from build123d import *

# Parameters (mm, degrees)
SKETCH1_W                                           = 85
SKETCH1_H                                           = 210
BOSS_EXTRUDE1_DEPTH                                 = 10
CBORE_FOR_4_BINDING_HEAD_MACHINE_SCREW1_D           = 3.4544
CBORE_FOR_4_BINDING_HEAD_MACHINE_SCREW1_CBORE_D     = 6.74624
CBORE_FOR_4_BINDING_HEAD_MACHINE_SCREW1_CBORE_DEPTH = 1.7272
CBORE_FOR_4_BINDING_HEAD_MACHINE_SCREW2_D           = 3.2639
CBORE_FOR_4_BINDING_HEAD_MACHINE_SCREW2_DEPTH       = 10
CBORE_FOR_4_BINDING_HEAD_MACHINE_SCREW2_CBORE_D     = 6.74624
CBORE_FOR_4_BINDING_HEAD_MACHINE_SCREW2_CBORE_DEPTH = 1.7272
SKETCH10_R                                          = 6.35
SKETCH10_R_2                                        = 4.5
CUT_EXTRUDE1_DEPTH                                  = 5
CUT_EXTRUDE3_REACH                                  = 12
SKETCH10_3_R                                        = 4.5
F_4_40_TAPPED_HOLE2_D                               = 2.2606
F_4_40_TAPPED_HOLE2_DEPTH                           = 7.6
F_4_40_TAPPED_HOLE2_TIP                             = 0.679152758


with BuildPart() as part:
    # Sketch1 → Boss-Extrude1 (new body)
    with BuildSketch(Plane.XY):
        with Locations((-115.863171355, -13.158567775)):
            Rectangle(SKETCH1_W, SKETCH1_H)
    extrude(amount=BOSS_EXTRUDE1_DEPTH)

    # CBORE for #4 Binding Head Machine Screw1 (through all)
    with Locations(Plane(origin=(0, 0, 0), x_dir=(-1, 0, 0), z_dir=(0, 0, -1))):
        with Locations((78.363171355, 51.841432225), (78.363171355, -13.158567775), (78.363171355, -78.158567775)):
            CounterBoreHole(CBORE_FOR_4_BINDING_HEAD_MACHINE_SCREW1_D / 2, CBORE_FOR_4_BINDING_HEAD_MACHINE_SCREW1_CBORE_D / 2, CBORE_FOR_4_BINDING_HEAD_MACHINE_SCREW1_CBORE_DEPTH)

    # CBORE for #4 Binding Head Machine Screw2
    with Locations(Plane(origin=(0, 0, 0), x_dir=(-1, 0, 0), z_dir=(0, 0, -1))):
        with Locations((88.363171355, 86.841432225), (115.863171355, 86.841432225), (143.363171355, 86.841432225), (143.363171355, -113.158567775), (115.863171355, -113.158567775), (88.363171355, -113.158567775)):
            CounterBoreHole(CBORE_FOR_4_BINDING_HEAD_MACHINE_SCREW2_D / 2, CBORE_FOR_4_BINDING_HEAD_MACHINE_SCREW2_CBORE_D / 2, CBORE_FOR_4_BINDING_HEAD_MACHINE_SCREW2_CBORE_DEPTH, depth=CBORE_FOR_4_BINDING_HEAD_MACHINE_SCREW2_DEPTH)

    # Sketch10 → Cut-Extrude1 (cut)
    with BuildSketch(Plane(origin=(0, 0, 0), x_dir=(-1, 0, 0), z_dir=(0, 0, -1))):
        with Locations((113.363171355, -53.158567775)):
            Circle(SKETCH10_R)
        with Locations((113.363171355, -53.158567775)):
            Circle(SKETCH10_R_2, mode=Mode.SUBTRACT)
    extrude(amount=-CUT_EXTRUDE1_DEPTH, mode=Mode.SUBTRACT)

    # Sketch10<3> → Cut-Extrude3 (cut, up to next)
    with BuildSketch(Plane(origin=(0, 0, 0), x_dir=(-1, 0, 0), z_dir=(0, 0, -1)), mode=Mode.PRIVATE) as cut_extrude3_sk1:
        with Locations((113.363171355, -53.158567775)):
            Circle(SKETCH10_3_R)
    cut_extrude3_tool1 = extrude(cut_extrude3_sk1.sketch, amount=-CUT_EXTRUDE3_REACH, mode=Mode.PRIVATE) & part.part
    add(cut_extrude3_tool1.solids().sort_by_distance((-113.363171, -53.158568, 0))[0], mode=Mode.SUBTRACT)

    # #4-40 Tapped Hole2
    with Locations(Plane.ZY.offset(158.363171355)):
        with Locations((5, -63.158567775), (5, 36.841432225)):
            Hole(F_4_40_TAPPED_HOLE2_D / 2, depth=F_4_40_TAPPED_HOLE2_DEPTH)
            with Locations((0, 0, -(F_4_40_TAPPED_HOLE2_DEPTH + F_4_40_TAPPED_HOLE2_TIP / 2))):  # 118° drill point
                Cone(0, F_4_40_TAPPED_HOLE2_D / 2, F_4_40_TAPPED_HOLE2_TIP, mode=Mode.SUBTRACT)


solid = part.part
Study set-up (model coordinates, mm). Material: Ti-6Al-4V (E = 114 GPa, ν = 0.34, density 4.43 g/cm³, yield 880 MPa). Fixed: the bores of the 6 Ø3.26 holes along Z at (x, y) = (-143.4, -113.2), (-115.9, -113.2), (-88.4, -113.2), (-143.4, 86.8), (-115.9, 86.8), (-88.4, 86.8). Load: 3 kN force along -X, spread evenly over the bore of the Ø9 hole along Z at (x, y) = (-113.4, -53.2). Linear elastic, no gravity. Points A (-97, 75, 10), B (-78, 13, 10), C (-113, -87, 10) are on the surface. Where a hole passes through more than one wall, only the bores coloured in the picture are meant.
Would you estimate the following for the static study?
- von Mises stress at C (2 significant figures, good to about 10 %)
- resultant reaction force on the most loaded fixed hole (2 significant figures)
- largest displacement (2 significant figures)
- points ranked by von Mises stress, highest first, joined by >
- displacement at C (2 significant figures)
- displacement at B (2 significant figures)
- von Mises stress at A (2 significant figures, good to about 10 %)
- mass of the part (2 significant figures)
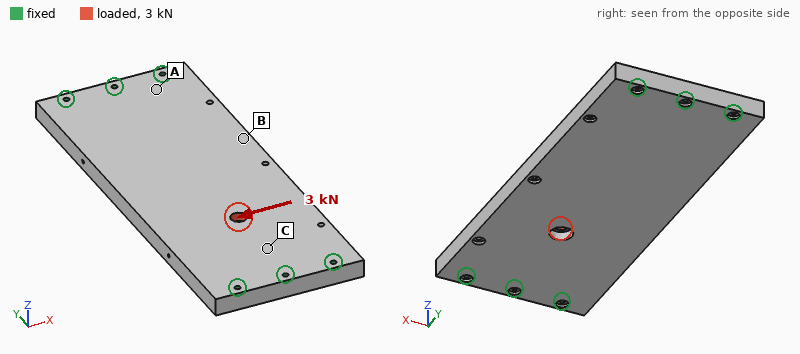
9.4 MPa
1.2 kN
11 µm
C > A > B
3.6 µm
7.1 µm
4.5 MPa
780 g
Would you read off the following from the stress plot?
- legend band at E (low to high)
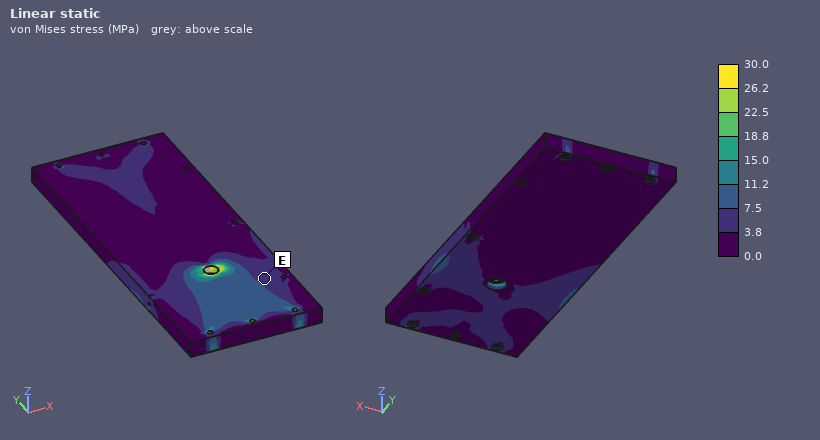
3.8 to 7.5 MPa
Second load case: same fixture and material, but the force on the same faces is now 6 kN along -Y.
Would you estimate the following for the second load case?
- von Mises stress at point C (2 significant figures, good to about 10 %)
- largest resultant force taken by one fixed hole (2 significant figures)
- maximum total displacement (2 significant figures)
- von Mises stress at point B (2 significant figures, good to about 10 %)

10 MPa
1.4 kN
12 µm
4.1 MPa
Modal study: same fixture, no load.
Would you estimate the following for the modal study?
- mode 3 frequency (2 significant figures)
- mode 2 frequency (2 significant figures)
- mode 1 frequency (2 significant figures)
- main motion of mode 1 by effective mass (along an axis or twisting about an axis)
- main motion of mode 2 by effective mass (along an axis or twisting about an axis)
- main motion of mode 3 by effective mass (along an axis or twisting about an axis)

3100 Hz
2100 Hz
1100 Hz
along Z
twisting about Y
twisting about X
